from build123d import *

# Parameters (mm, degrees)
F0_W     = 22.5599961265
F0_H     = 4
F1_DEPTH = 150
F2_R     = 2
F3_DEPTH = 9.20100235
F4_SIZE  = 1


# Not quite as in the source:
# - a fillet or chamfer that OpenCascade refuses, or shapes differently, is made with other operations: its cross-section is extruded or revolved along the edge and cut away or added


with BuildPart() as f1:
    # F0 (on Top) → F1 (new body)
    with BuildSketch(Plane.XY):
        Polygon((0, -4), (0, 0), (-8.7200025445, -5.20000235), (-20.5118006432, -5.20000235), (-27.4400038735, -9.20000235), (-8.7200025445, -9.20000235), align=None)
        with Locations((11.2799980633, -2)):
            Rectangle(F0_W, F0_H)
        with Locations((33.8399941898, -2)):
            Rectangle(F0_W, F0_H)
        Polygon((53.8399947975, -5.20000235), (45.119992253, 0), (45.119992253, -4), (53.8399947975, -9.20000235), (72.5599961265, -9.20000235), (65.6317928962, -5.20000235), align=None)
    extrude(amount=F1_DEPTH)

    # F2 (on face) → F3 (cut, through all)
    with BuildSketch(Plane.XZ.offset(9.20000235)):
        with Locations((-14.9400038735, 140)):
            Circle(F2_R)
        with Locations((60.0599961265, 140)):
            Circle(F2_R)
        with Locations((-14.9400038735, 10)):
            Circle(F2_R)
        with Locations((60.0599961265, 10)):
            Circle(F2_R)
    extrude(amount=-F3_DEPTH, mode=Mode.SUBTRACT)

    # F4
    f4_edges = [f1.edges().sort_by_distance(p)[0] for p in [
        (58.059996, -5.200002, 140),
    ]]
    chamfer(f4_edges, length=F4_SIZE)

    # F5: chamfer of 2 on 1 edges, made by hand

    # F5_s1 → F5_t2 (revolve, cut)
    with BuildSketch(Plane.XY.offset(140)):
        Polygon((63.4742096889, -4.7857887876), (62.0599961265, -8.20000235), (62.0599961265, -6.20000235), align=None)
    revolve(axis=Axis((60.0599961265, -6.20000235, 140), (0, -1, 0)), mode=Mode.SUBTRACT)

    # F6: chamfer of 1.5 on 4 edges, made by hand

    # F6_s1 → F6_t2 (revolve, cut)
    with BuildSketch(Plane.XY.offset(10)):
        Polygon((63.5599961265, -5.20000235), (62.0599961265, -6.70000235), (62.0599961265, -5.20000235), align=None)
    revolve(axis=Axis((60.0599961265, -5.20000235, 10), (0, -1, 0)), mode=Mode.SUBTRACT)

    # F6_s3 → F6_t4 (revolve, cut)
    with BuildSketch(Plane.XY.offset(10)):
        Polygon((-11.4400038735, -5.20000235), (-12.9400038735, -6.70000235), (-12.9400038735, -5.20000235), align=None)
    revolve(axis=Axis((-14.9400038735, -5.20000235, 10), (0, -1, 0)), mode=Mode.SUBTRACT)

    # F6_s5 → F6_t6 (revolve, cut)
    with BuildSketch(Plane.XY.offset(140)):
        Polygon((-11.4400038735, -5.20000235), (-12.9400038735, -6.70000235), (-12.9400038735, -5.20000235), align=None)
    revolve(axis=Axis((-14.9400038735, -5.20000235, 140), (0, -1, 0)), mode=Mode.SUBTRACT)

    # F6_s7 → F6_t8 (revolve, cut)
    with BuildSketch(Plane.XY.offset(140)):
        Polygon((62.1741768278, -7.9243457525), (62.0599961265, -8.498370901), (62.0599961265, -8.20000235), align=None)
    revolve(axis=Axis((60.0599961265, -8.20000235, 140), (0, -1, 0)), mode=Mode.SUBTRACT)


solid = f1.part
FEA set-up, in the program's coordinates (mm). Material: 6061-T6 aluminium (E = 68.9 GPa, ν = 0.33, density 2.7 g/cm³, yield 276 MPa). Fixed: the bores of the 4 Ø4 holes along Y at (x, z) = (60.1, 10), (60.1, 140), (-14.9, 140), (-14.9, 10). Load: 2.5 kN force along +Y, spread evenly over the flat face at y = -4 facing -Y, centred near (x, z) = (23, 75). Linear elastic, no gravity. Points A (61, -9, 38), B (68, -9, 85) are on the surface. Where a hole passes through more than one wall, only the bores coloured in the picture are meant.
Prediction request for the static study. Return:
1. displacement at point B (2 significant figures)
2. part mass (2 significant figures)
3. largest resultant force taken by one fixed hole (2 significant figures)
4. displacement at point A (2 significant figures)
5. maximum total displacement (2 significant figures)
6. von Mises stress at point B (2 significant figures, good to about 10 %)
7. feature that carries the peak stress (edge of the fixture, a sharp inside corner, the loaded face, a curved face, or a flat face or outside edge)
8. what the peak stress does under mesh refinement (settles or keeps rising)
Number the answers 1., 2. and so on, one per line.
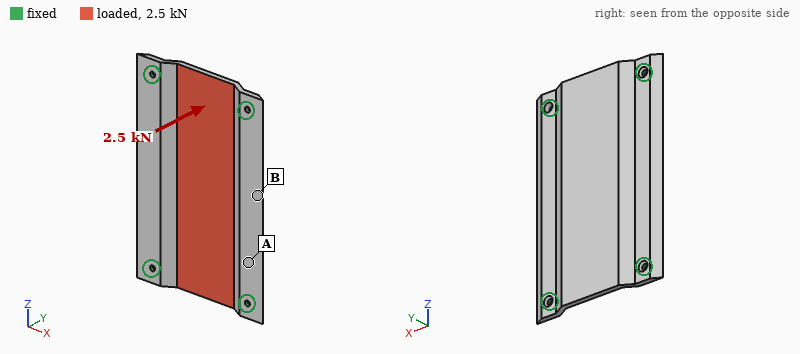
1. 0.17 mm
2. 150 g
3. 2.3 kN
4. 0.098 mm
5. 0.23 mm
6. 25 MPa
7. edge of the fixture
8. keeps rising
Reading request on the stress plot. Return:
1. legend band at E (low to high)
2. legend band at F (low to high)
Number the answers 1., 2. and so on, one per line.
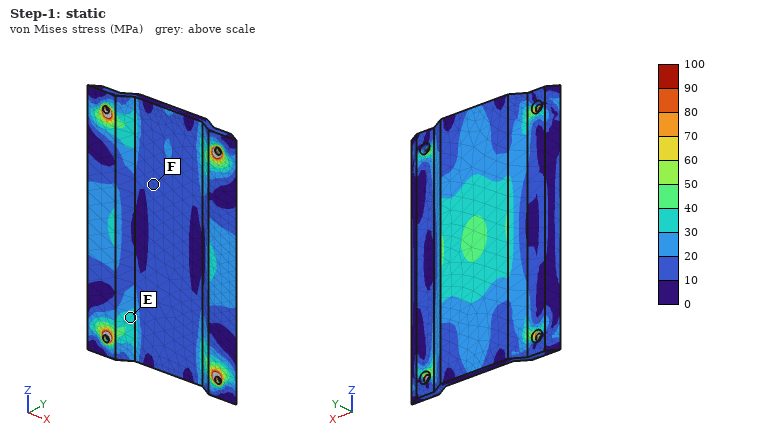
1. 30 to 40 MPa
2. 10 to 20 MPa
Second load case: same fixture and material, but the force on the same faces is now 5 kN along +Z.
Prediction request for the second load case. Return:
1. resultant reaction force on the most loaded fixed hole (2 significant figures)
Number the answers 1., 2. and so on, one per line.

1. 1.4 kN
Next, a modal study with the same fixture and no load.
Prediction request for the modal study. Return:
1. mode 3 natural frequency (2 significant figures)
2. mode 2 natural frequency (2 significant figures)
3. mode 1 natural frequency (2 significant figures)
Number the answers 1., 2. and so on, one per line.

1. 3300 Hz
2. 1600 Hz
3. 1500 Hz
